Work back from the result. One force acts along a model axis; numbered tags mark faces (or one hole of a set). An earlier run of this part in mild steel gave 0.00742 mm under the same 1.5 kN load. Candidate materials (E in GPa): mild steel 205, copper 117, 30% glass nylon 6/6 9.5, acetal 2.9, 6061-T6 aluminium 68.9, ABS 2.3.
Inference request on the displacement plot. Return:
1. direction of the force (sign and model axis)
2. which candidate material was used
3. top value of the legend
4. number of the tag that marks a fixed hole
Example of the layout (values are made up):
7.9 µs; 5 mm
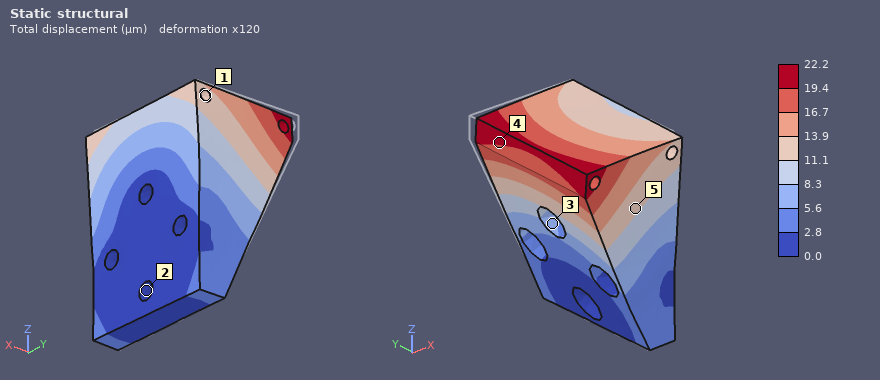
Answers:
-Y; 6061-T6 aluminium; 22.2 µm; 2
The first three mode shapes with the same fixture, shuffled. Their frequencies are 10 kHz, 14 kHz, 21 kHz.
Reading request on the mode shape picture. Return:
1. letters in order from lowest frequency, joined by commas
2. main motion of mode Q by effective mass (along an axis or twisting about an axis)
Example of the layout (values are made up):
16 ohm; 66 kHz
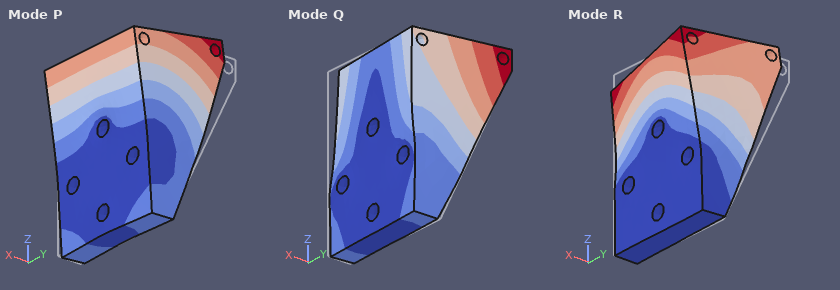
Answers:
P, Q, R; along Y
